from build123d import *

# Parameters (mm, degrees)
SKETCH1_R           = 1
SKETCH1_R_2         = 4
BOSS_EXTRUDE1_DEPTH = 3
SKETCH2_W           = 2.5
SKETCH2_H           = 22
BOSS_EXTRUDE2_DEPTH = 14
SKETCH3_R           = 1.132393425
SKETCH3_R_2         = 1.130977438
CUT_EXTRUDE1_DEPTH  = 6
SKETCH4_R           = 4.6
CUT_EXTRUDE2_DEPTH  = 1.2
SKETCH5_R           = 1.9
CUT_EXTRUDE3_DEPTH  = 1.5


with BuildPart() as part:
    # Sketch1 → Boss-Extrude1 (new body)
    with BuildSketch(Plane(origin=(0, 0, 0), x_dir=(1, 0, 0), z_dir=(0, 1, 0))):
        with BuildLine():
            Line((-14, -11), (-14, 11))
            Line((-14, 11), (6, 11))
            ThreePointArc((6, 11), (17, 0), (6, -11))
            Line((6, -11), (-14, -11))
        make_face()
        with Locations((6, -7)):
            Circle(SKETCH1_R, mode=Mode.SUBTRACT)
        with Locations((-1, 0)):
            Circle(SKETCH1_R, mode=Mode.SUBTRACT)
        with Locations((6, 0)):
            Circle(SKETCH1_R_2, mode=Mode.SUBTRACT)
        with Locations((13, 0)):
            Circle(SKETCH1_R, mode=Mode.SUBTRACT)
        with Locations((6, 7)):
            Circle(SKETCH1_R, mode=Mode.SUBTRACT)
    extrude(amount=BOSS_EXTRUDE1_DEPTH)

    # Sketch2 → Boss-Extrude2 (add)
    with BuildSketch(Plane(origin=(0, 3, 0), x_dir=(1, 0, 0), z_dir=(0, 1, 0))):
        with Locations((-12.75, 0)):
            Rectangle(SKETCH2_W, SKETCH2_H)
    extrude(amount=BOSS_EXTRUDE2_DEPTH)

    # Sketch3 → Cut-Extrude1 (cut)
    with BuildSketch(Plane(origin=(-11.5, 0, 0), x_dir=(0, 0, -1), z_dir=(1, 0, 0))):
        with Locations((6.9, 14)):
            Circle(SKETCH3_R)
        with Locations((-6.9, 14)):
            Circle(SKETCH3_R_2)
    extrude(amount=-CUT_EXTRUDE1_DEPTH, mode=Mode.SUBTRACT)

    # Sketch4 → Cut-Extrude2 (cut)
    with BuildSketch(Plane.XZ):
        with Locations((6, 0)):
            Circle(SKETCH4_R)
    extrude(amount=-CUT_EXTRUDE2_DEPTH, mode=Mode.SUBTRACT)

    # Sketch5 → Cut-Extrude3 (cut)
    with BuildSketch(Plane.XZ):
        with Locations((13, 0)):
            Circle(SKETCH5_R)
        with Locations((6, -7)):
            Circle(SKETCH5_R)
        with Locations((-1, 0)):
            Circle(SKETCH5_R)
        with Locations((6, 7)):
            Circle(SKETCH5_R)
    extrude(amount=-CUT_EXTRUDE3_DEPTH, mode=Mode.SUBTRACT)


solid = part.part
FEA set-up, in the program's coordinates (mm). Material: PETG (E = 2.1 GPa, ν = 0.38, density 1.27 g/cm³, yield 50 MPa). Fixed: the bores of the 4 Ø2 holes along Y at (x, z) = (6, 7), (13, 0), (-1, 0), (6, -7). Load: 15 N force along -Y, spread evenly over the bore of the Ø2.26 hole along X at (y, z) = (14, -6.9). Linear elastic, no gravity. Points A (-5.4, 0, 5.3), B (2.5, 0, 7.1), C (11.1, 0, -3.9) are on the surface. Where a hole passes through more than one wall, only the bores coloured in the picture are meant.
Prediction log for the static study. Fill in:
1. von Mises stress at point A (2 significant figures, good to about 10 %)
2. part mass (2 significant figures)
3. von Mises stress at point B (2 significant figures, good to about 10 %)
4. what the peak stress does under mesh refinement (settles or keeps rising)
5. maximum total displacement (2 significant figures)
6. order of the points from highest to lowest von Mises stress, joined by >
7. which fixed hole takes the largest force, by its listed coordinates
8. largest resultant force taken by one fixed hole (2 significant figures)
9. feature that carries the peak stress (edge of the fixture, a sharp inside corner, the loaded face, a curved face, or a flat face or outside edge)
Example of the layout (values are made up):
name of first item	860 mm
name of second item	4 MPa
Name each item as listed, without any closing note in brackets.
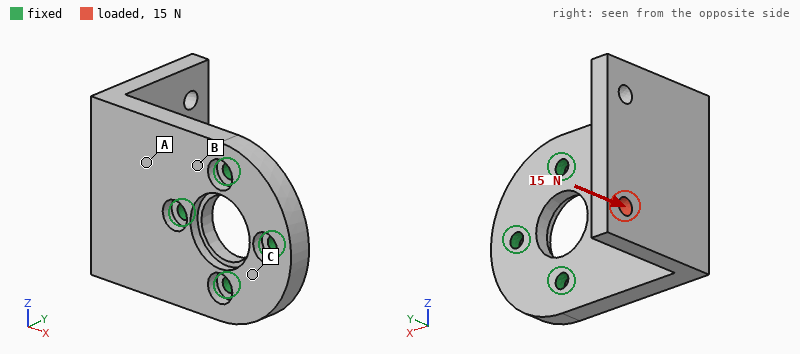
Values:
von Mises stress at point A	4.9 MPa
part mass	3.0 g
von Mises stress at point B	2.3 MPa
what the peak stress does under mesh refinement	keeps rising
maximum total displacement	0.42 mm
order of the points from highest to lowest von Mises stress, joined by >	A > B > C
which fixed hole takes the largest force, by its listed coordinates	(-1, 0)
largest resultant force taken by one fixed hole	34 N
feature that carries the peak stress	edge of the fixture
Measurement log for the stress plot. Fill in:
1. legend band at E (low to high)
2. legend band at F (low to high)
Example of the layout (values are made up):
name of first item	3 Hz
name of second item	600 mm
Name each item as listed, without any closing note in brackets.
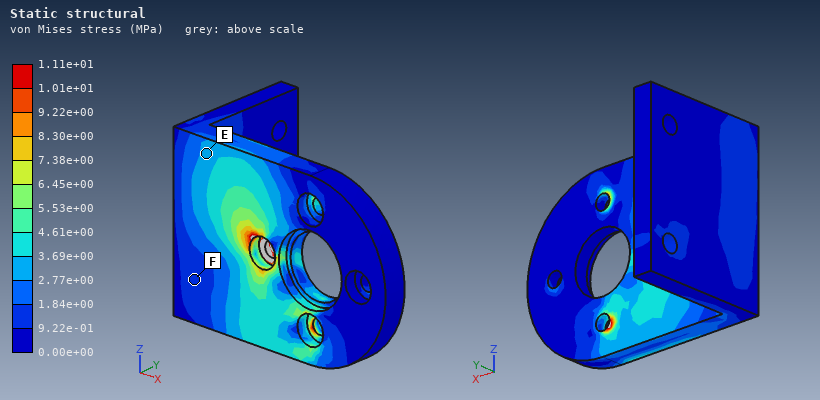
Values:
legend band at E	2.77e+00 to 3.69e+00 MPa
legend band at F	9.22e-01 to 1.84e+00 MPa
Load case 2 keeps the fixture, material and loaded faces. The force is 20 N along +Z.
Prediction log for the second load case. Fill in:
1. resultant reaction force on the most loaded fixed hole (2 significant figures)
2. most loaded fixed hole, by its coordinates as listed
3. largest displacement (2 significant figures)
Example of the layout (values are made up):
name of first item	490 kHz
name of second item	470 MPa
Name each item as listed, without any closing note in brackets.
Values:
resultant reaction force on the most loaded fixed hole	29 N
most loaded fixed hole, by its coordinates as listed	(-1, 0)
largest displacement	0.49 mm
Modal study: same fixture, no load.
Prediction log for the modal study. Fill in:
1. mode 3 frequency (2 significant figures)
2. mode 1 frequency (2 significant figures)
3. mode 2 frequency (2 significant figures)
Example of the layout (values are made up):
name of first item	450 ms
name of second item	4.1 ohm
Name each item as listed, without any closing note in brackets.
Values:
mode 3 frequency	2400 Hz
mode 1 frequency	1000 Hz
mode 2 frequency	1300 Hz
